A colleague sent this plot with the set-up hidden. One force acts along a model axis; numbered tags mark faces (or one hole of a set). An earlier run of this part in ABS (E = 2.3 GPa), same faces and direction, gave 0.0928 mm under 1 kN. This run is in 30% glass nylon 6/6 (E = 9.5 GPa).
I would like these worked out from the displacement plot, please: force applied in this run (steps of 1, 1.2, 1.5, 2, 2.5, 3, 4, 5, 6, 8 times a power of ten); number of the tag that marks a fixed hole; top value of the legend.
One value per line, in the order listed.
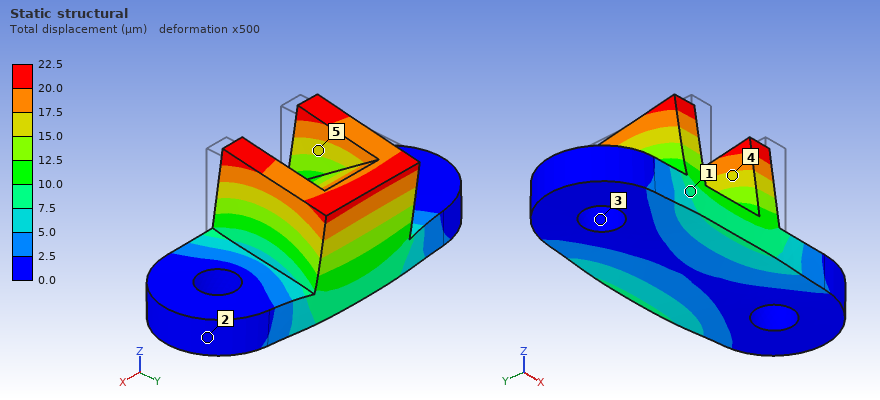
1 kN
3
22.5 µm
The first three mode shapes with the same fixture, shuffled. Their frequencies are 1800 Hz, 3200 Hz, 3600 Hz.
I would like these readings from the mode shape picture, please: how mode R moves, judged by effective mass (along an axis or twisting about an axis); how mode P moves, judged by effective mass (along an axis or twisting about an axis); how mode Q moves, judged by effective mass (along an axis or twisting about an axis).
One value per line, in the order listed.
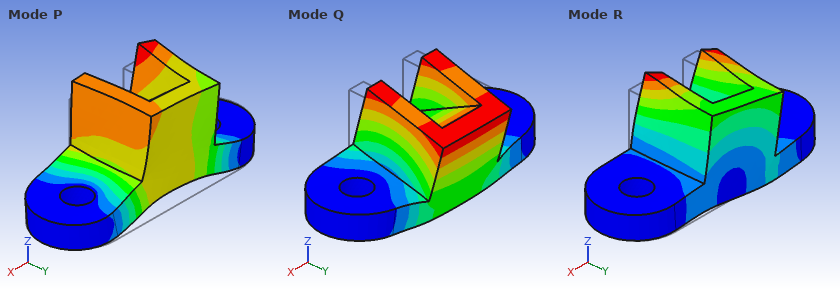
along X
along Z
along Y
